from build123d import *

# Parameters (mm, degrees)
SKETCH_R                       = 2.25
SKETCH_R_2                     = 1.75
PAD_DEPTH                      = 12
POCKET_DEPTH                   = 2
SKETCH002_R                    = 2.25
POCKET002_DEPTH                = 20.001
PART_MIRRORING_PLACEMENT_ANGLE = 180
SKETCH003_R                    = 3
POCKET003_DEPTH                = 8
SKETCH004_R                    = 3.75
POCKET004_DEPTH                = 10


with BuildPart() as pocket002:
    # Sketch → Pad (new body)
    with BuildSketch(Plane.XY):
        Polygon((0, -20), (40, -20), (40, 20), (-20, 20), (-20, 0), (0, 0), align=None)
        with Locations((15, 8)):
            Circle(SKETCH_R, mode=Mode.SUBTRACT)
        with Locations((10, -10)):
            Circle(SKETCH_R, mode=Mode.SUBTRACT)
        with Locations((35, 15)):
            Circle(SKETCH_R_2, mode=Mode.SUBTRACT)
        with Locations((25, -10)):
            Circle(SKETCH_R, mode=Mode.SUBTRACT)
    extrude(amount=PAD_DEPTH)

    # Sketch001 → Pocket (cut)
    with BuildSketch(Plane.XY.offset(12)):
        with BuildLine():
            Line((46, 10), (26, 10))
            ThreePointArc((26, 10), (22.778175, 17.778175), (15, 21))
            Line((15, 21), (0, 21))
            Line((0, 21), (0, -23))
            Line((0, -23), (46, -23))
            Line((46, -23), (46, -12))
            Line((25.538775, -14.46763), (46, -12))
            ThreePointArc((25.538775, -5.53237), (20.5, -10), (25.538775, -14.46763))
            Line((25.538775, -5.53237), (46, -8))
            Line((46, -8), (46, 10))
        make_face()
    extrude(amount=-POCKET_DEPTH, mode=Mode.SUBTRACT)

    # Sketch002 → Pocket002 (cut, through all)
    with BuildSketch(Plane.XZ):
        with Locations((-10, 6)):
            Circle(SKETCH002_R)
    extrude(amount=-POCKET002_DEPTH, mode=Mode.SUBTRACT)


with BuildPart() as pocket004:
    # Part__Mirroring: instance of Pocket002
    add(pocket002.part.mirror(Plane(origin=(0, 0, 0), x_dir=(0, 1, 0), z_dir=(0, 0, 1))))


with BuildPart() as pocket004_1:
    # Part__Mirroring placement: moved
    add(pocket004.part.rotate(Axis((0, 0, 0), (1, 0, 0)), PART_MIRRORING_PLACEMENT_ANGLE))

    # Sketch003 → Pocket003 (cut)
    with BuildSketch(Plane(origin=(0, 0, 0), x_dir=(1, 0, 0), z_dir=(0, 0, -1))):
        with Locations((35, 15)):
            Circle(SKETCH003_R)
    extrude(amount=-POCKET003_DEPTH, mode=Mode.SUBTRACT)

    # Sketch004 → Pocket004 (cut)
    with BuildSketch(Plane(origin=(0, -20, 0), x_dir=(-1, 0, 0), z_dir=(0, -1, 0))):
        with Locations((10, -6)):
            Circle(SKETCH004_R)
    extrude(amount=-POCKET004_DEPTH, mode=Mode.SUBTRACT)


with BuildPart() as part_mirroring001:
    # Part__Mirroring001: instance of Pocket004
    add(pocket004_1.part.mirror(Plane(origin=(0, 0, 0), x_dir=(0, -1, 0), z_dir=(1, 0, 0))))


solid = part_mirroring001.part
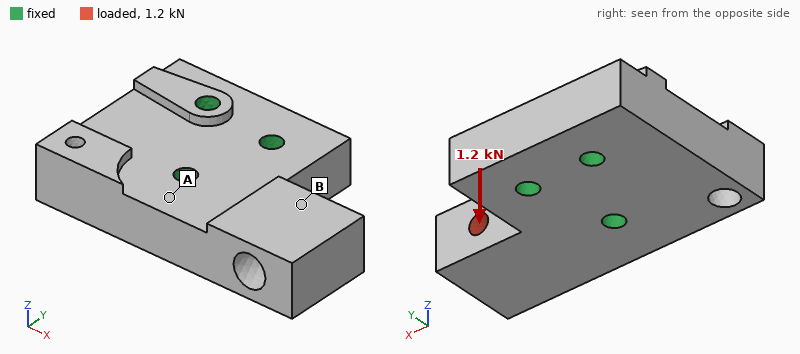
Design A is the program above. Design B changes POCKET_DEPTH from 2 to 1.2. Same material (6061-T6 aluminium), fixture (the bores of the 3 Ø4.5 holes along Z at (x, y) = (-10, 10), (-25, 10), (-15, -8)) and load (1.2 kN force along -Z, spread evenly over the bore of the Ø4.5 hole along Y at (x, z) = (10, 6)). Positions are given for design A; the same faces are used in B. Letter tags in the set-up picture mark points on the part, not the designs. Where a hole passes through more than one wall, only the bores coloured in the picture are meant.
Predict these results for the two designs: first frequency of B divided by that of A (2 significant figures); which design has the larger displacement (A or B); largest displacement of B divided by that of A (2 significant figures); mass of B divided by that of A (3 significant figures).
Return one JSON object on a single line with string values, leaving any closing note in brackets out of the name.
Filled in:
{"first frequency of B divided by that of A": "1.1", "which design has the larger displacement": "A", "largest displacement of B divided by that of A": "0.83", "mass of B divided by that of A": "1.05"}
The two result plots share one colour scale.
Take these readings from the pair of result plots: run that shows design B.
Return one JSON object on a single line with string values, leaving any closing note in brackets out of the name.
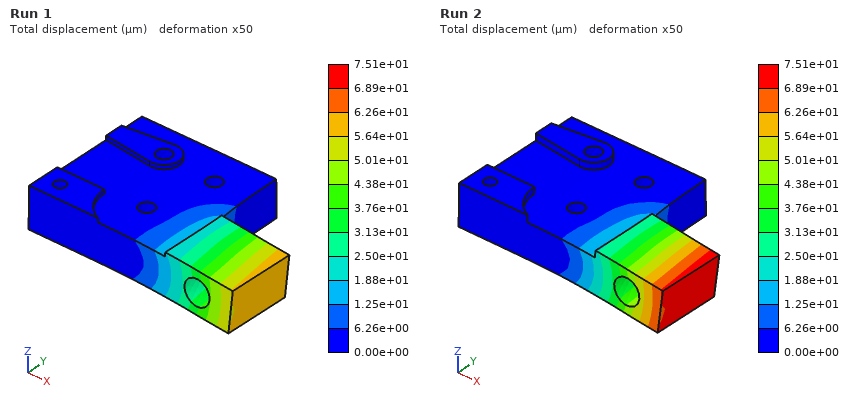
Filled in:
{"run that shows design B": "Run 1"}
